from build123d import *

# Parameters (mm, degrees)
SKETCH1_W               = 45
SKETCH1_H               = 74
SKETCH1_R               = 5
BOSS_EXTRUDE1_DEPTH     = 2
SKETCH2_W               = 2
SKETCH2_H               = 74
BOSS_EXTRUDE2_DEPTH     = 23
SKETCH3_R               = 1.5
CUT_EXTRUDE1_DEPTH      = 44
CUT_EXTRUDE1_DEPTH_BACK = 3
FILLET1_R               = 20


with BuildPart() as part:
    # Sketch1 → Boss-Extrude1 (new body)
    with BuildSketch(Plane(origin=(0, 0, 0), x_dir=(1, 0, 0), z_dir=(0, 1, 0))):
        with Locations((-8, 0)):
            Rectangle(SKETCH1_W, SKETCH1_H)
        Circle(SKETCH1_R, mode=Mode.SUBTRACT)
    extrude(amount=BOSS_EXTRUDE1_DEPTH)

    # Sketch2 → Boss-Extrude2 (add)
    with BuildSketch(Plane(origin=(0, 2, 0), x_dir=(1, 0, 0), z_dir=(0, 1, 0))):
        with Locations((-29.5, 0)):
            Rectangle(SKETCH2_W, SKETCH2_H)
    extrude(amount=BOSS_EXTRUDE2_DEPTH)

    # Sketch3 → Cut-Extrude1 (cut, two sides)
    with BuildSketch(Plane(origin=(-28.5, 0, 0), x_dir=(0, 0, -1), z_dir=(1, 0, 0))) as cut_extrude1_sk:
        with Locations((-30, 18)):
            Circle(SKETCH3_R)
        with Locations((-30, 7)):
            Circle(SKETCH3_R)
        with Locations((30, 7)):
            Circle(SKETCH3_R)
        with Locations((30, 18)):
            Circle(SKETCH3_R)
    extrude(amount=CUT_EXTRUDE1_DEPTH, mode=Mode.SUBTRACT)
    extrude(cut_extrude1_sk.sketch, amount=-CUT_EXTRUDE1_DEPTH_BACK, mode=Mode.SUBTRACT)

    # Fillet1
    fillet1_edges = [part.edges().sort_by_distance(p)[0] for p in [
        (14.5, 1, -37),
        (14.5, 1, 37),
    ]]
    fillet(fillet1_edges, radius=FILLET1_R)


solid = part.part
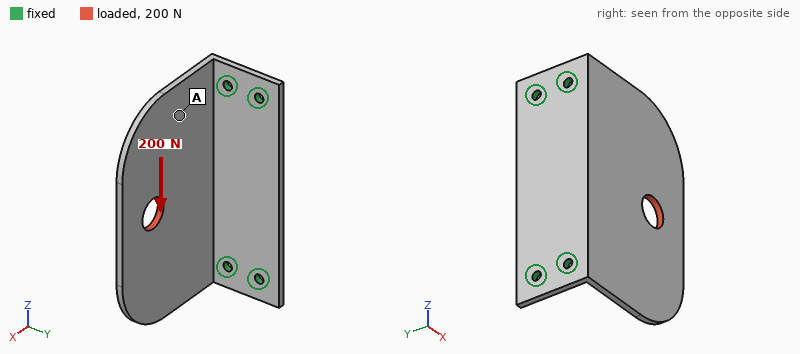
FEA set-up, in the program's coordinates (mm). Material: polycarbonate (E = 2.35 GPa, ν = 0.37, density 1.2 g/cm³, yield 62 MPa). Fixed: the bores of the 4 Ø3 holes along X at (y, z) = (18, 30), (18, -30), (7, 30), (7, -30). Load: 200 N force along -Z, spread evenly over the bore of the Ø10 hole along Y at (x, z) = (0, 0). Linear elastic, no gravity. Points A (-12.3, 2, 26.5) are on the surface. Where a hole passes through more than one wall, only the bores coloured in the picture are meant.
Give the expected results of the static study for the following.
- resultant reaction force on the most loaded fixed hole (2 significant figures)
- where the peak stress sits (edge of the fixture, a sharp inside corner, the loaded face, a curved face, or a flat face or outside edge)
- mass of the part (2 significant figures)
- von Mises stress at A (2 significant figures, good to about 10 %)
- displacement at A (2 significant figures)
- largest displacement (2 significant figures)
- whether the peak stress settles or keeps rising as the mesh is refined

130 N
edge of the fixture
11 g
4.3 MPa
0.50 mm
0.92 mm
keeps rising
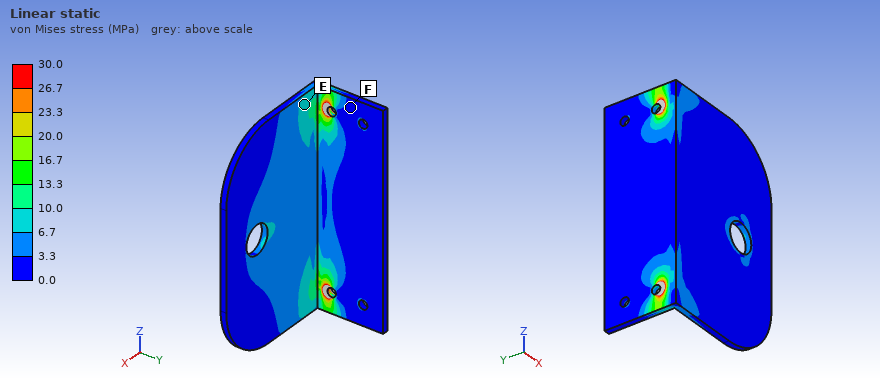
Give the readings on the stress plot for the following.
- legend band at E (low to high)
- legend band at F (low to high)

6.7 to 10.0 MPa
0.0 to 3.3 MPa
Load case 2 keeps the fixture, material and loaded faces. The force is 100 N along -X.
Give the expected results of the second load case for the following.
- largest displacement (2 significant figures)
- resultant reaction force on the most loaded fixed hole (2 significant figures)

0.91 mm
62 N
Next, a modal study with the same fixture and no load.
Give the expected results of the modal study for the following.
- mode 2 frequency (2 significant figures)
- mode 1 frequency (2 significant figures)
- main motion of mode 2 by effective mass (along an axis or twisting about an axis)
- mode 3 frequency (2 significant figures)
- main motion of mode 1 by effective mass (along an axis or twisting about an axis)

420 Hz
200 Hz
twisting about X
900 Hz
along Y
